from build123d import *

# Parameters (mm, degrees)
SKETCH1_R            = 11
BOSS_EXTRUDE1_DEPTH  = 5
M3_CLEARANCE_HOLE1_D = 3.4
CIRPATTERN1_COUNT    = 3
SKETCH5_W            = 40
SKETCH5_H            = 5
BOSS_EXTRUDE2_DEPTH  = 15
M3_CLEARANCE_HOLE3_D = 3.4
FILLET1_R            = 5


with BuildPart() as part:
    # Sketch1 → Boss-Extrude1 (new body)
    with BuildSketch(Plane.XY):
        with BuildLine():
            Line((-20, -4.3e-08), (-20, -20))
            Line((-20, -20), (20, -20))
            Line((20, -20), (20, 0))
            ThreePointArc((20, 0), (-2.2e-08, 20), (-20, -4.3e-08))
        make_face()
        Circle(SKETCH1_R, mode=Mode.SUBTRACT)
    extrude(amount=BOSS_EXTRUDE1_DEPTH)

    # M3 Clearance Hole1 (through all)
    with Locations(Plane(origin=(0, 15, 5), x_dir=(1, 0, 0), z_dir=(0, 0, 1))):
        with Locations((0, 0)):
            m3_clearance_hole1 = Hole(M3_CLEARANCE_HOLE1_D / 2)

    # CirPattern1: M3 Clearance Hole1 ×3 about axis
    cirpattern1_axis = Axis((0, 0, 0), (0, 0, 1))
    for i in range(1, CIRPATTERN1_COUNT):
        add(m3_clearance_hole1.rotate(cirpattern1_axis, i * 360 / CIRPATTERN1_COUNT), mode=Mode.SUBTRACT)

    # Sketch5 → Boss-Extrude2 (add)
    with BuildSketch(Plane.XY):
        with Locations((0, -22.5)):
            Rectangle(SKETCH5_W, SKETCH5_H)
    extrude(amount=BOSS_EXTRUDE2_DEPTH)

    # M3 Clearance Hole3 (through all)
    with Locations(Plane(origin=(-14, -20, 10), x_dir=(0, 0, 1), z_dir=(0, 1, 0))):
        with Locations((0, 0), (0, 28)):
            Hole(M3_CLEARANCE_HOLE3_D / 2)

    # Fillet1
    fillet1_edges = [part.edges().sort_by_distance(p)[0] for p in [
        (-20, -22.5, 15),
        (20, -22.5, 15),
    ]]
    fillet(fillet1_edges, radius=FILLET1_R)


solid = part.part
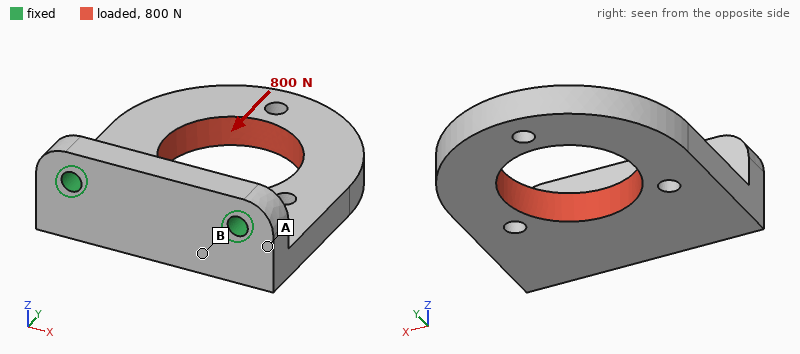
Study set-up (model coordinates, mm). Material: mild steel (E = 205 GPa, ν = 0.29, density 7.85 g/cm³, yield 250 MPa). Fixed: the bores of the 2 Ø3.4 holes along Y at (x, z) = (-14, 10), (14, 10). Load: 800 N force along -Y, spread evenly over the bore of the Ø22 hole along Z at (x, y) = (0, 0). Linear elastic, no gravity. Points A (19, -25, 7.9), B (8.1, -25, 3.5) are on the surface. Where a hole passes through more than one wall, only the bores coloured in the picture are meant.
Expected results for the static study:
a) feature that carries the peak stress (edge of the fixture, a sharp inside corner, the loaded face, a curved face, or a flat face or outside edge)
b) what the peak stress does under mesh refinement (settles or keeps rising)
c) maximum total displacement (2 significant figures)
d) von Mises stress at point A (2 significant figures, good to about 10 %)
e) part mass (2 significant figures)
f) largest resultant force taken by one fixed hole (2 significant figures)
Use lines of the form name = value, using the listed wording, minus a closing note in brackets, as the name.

feature that carries the peak stress = edge of the fixture
what the peak stress does under mesh refinement = keeps rising
maximum total displacement = 17 µm
von Mises stress at point A = 21 MPa
part mass = 62 g
largest resultant force taken by one fixed hole = 400 N
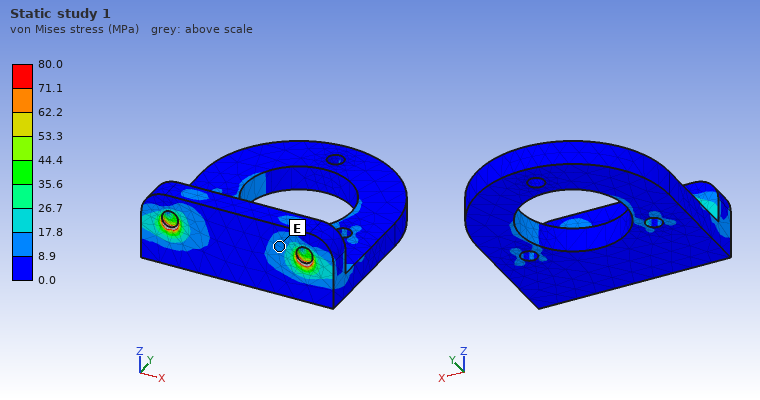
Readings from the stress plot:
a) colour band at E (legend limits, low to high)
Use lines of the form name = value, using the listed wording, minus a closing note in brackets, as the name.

colour band at E = 8.9 to 17.8 MPa
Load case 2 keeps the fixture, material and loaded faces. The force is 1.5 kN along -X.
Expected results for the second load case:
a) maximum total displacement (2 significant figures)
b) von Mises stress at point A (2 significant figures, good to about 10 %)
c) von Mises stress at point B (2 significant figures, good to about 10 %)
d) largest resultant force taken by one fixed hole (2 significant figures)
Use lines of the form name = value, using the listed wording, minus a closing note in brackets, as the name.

maximum total displacement = 28 µm
von Mises stress at point A = 44 MPa
von Mises stress at point B = 23 MPa
largest resultant force taken by one fixed hole = 1.4 kN
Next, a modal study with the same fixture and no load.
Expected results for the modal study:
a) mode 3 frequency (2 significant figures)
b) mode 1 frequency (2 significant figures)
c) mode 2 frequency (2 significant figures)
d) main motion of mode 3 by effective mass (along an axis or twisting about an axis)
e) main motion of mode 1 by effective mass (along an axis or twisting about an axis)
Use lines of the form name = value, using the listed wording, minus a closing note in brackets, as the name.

mode 3 frequency = 7600 Hz
mode 1 frequency = 2100 Hz
mode 2 frequency = 5500 Hz
main motion of mode 3 by effective mass = along X
main motion of mode 1 by effective mass = along Z
